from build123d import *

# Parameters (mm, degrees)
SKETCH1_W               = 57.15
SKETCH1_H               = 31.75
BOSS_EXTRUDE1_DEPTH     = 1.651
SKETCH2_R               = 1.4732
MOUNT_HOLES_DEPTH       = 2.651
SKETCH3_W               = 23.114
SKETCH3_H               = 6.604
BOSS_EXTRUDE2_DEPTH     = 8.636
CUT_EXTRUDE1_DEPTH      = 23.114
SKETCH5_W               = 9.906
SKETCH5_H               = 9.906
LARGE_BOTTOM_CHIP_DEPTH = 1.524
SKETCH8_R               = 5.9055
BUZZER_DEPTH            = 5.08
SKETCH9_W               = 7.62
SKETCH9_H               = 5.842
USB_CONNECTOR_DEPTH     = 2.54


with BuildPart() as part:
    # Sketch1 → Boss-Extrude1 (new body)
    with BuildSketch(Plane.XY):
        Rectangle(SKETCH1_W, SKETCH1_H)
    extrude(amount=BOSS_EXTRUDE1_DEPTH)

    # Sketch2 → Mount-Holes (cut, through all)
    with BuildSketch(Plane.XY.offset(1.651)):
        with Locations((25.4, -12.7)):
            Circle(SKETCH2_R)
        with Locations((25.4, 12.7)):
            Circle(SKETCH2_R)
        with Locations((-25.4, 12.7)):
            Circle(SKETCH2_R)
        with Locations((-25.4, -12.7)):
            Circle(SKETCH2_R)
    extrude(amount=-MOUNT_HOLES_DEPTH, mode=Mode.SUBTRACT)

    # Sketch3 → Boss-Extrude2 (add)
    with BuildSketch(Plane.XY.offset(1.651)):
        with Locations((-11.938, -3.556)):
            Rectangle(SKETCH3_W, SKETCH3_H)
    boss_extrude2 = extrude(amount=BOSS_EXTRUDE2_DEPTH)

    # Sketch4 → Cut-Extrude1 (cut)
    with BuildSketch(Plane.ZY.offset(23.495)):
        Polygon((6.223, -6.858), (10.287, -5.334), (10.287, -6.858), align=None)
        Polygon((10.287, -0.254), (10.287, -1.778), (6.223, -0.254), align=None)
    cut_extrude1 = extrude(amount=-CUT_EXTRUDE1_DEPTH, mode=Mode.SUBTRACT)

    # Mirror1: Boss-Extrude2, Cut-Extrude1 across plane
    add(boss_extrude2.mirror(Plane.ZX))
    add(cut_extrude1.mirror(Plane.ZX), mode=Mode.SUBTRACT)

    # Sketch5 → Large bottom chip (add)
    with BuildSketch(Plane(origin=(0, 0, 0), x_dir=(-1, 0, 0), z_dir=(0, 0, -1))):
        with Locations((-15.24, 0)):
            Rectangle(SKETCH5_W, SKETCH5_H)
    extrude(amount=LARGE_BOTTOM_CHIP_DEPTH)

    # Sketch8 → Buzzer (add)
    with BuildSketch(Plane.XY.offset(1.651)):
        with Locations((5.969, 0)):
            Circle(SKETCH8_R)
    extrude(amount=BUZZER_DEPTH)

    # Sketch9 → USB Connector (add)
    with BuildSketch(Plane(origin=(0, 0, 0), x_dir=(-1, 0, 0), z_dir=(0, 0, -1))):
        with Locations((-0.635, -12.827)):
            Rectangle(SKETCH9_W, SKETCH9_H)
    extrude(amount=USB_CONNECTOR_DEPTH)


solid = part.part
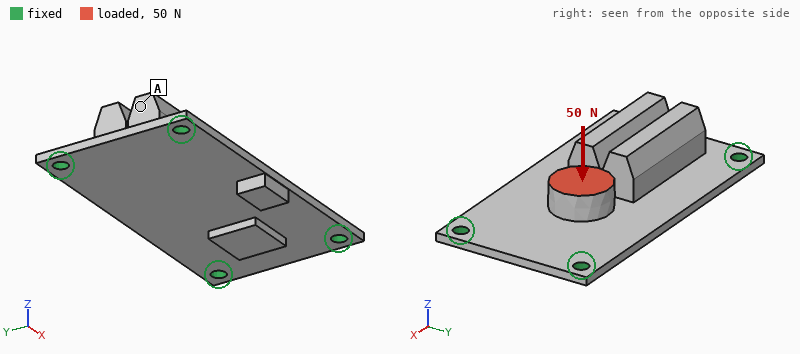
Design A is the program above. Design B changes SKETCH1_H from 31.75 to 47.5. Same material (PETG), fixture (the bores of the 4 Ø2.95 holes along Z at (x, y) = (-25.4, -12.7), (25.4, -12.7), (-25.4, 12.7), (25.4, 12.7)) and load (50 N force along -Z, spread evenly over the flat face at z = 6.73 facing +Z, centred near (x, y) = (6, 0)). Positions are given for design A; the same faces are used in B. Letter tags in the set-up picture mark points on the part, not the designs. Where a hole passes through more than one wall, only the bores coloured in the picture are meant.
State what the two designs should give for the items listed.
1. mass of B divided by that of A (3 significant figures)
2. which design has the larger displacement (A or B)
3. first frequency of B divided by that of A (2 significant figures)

1.24
A
1.0
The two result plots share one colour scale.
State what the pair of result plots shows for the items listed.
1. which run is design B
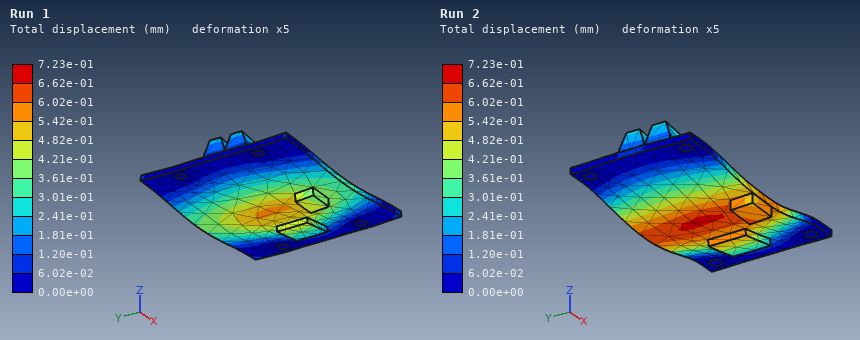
Run 1
